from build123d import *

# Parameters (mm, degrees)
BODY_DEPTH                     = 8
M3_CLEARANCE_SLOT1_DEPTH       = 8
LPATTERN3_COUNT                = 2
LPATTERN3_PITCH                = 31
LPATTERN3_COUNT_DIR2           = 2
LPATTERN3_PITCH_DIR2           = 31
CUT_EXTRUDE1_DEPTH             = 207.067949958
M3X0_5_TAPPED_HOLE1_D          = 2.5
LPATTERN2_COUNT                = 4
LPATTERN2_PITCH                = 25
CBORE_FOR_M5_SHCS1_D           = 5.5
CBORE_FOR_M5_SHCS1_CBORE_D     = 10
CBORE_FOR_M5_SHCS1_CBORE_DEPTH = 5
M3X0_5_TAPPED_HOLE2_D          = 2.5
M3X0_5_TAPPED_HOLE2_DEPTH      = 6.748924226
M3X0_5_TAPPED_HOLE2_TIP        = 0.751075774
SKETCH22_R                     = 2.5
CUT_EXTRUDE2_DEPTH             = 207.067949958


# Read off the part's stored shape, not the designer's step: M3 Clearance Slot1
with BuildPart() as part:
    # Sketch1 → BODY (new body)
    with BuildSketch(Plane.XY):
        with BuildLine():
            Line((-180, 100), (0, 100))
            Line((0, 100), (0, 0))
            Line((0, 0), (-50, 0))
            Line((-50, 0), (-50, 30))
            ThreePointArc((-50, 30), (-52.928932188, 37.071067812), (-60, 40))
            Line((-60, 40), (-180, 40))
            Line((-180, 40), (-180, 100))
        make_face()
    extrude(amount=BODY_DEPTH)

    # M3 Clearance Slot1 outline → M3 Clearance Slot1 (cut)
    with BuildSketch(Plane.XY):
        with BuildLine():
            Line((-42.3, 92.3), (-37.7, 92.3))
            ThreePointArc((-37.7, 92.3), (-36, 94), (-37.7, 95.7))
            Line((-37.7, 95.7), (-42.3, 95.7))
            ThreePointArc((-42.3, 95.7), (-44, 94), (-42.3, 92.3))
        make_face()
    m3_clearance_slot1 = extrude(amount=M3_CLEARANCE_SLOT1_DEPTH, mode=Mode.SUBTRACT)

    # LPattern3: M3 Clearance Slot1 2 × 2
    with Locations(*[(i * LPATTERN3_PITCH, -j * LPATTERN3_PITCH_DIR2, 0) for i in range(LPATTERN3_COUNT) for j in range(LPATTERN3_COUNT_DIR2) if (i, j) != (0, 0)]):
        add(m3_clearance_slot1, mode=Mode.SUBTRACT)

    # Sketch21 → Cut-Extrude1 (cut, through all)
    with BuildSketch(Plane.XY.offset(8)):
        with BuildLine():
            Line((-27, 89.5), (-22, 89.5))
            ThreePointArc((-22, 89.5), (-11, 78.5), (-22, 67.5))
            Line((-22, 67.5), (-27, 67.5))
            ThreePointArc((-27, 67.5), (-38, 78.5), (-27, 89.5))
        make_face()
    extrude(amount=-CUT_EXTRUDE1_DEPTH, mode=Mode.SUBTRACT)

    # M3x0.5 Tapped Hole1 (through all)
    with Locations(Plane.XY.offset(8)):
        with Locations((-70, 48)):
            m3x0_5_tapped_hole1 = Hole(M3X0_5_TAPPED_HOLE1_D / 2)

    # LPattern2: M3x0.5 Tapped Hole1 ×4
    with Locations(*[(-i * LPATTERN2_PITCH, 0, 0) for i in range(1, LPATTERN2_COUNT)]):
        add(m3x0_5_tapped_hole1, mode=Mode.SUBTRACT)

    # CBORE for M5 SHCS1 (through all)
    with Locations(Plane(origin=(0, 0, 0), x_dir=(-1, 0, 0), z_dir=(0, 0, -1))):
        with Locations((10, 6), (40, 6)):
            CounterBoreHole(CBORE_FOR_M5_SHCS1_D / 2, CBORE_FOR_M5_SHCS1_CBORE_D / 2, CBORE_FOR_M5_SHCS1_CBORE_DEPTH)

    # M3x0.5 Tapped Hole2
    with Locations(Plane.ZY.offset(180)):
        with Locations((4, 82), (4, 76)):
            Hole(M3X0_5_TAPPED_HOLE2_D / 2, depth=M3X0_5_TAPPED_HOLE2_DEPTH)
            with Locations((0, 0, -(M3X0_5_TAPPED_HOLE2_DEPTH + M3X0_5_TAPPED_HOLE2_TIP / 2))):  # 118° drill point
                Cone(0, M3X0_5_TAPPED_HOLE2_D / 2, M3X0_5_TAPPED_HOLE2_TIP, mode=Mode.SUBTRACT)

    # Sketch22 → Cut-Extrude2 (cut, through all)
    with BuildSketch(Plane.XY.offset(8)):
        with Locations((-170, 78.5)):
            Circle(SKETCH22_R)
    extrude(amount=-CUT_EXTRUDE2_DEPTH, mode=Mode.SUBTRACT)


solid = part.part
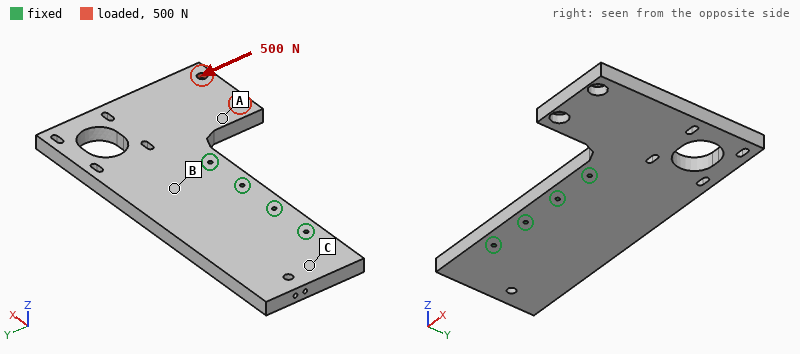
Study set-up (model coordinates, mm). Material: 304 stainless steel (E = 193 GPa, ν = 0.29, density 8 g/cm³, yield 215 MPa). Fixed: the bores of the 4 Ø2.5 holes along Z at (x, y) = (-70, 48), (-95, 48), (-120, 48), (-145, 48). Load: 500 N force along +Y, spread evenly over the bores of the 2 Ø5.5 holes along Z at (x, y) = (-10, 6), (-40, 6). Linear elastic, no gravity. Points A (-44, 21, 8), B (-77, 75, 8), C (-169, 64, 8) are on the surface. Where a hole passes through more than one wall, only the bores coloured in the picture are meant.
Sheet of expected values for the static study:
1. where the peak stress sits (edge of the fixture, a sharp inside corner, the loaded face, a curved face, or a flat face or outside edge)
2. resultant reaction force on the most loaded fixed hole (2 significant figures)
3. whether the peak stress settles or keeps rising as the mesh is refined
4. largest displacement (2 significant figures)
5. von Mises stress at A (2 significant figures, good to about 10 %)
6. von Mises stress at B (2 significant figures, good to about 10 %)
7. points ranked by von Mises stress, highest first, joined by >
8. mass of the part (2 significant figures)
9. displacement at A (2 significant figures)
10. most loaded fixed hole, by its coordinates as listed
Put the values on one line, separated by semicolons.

edge of the fixture; 840 N; keeps rising; 12 µm; 4.2 MPa; 1.8 MPa; A > B > C; 770 g; 5.6 µm; (-70, 48)
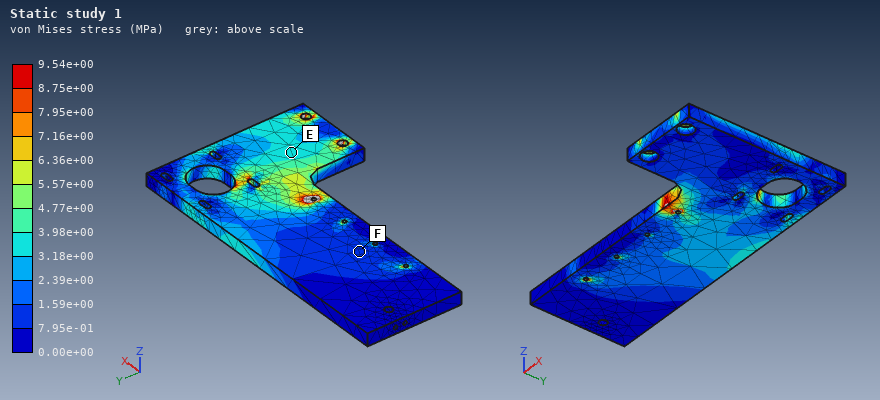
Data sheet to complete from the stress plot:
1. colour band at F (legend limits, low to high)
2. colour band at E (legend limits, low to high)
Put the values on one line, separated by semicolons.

7.95e-01 to 1.59e+00 MPa; 3.18e+00 to 3.98e+00 MPa
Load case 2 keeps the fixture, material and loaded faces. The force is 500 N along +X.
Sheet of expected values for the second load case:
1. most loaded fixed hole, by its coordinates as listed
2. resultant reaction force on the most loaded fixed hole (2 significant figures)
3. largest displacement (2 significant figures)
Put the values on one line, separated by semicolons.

(-70, 48); 780 N; 15 µm
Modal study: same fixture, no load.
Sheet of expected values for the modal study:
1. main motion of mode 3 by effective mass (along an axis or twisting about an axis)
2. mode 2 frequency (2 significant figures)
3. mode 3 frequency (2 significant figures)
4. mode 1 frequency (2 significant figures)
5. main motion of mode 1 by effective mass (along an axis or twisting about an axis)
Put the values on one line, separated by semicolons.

along Z; 1100 Hz; 1800 Hz; 810 Hz; along Z
